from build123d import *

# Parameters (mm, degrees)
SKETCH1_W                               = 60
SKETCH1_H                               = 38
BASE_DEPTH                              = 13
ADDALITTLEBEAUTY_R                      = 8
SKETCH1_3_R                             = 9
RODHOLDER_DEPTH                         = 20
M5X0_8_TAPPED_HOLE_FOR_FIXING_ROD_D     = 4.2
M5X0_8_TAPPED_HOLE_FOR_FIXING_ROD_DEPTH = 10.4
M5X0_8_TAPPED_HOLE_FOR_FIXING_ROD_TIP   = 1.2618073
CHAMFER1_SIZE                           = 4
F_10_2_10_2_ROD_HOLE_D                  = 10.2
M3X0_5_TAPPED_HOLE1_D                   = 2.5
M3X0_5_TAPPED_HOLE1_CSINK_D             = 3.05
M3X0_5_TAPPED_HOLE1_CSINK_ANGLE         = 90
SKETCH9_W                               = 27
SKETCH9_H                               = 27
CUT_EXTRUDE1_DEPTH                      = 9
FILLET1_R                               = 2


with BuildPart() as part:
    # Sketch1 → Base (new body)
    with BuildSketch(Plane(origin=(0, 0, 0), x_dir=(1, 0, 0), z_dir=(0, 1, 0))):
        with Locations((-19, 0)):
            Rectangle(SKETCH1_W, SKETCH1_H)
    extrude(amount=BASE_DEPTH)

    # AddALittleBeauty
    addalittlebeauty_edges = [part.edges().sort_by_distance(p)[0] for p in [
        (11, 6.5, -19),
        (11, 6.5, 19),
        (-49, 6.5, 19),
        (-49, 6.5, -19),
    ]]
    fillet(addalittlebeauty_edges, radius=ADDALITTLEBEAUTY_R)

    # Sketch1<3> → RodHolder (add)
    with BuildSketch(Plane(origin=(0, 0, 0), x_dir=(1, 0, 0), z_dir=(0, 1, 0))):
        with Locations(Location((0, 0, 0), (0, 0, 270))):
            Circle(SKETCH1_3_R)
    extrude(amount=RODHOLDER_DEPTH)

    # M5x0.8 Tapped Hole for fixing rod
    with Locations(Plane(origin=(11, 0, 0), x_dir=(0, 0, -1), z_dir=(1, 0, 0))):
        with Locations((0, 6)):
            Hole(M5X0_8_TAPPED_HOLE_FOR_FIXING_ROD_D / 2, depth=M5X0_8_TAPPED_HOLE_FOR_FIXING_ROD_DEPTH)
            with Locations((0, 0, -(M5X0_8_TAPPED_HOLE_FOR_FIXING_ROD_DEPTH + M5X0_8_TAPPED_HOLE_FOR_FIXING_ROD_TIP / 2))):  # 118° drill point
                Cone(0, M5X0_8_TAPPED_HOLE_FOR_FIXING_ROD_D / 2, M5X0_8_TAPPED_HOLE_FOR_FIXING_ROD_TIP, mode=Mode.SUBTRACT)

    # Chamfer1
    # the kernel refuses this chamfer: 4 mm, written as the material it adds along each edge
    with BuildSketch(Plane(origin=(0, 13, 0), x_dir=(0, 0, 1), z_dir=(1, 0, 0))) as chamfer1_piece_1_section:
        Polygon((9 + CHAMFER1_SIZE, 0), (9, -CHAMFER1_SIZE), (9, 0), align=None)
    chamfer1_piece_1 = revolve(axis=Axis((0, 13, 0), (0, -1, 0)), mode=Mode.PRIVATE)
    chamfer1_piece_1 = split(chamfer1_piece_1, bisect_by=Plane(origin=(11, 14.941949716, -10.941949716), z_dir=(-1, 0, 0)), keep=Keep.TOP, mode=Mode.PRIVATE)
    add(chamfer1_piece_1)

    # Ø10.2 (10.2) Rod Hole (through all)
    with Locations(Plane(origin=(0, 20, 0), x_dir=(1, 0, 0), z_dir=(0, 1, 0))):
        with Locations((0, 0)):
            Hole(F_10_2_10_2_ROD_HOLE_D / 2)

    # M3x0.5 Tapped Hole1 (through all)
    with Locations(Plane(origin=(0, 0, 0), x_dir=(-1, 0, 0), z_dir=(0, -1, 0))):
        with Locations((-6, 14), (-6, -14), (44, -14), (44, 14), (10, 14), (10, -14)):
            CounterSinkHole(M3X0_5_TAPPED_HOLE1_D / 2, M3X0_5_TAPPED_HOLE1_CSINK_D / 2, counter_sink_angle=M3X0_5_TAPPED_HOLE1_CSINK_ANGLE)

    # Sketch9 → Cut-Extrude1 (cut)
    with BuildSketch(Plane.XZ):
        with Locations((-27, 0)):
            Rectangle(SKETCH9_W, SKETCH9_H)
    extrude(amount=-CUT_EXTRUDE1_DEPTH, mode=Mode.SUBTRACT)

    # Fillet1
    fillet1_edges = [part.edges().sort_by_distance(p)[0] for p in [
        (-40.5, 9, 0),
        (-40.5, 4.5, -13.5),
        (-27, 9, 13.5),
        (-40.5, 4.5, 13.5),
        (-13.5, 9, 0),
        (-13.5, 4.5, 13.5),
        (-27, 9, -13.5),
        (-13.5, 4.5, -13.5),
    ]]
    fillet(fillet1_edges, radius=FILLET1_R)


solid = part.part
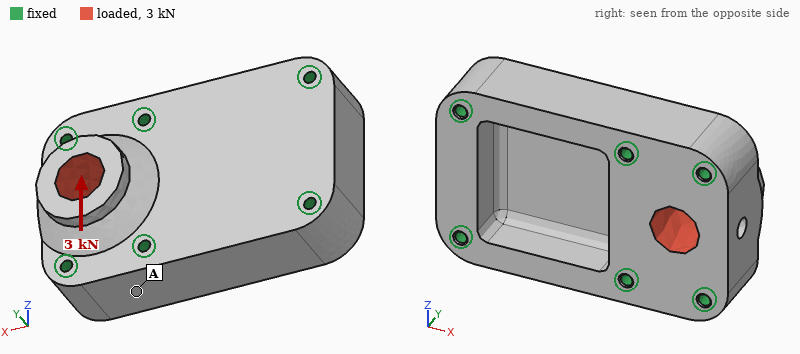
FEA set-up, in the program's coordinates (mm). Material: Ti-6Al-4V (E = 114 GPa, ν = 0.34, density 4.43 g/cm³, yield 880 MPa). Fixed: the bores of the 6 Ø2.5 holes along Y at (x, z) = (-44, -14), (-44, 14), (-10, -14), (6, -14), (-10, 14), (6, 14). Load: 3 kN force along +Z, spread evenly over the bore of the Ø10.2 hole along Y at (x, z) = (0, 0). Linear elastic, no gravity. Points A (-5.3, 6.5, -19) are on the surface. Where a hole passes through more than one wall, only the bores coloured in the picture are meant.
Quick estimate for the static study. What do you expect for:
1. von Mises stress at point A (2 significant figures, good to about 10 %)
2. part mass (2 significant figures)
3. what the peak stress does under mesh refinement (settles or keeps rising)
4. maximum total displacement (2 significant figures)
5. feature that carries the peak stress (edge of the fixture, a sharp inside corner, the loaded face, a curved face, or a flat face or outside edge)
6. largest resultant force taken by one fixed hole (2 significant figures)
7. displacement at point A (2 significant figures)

2.6 MPa
100 g
keeps rising
1.6 µm
edge of the fixture
880 N
0.30 µm
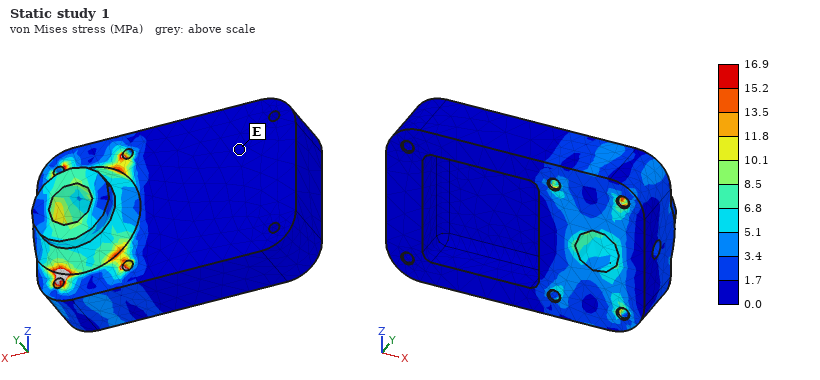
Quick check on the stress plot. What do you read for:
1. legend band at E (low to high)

0.0 to 1.7 MPa
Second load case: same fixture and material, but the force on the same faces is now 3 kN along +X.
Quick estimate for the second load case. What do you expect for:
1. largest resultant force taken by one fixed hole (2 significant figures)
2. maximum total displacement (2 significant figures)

860 N
2.9 µm
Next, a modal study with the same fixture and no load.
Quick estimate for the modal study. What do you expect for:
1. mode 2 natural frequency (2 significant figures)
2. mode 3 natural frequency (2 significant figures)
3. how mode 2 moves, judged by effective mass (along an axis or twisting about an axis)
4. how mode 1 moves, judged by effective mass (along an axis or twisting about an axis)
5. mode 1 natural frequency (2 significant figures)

32 kHz
34 kHz
along Z
along Y
26 kHz
